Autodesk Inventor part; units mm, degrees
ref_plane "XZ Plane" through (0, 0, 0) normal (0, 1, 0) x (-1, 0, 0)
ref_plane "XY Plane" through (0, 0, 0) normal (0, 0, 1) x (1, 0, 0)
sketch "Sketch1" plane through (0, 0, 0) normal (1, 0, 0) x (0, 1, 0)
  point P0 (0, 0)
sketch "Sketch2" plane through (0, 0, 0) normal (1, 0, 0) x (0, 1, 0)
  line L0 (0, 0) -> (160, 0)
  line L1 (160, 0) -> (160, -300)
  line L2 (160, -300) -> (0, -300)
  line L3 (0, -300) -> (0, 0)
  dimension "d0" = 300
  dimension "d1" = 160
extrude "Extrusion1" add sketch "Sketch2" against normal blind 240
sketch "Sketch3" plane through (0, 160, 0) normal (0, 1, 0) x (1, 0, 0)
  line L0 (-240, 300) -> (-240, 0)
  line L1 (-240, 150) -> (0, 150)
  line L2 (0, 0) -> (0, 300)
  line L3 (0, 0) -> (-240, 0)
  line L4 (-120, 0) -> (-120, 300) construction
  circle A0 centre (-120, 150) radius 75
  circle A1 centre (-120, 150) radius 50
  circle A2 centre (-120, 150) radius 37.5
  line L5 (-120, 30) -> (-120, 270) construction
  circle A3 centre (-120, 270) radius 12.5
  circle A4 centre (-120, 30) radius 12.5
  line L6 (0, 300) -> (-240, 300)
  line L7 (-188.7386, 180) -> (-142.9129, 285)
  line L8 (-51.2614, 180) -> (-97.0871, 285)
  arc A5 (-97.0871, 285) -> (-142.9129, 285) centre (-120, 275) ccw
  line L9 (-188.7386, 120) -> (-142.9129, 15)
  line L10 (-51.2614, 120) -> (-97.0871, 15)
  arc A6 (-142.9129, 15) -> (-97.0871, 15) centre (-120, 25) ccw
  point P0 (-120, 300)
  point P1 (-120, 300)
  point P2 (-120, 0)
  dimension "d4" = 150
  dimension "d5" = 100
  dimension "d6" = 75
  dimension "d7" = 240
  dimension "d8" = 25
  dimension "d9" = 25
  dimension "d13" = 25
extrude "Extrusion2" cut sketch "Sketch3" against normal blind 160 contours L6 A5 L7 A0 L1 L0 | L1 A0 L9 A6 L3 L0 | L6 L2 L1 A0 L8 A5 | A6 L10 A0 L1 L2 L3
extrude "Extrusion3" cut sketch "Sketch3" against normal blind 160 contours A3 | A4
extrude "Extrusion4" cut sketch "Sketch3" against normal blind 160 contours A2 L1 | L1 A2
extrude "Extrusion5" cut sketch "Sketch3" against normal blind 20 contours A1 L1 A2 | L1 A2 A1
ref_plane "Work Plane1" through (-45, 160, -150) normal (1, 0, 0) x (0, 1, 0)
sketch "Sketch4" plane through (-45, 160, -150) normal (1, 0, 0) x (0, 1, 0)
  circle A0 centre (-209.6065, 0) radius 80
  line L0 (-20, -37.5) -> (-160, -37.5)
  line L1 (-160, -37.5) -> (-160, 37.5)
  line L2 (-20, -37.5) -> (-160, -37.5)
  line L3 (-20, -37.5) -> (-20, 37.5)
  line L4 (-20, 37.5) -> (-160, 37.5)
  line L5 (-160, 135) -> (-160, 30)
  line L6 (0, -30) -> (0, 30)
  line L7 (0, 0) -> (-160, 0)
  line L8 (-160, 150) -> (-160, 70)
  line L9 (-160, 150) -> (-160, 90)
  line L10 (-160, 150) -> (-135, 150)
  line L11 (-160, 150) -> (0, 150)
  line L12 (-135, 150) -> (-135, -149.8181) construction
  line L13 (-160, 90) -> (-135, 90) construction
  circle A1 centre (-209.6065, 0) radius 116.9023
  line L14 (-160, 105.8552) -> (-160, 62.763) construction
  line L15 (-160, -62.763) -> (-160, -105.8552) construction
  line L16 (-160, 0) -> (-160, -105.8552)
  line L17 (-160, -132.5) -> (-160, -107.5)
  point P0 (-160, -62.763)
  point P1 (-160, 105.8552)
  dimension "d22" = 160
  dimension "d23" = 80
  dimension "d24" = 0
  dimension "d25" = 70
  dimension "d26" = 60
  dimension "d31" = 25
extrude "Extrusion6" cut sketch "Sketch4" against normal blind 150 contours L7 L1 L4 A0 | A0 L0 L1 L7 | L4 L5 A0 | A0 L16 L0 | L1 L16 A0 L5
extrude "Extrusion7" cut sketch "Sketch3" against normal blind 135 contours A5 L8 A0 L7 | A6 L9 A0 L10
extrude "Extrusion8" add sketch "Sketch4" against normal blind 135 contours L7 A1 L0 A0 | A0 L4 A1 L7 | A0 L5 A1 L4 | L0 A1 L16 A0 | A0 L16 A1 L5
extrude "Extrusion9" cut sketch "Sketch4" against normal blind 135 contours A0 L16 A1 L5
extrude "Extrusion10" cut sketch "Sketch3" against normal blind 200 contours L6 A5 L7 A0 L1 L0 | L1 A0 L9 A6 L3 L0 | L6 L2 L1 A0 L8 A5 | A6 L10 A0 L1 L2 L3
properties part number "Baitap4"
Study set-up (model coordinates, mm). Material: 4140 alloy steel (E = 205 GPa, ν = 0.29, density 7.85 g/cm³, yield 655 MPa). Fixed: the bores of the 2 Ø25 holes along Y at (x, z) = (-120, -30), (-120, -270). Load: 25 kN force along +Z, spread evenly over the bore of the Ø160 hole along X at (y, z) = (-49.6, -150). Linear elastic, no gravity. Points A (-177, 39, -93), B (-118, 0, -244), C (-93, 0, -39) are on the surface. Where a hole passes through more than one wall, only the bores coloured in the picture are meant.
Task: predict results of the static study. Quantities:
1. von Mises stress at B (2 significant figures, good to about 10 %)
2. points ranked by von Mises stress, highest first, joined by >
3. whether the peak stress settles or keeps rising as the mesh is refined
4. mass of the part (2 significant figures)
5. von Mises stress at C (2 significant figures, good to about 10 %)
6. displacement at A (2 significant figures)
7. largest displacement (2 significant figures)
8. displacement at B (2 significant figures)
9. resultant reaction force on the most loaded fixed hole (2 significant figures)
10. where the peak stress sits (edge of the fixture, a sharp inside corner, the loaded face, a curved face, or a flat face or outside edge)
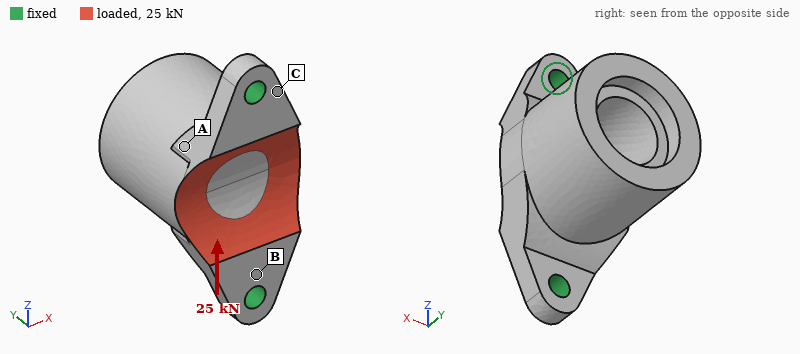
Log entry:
6.8 MPa
B > C > A
keeps rising
18 kg
3.5 MPa
2.8 µm
3.4 µm
0.51 µm
13 kN
edge of the fixture
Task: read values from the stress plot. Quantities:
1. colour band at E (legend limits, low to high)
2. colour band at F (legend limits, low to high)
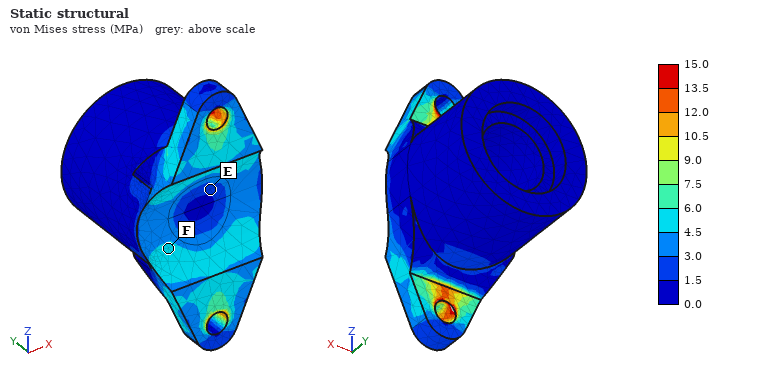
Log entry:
1.5 to 3.0 MPa
4.5 to 6.0 MPa
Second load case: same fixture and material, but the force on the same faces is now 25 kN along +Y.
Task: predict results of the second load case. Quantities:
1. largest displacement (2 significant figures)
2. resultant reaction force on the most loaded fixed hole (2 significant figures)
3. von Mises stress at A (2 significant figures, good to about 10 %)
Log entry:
11 µm
17 kN
5.3 MPa
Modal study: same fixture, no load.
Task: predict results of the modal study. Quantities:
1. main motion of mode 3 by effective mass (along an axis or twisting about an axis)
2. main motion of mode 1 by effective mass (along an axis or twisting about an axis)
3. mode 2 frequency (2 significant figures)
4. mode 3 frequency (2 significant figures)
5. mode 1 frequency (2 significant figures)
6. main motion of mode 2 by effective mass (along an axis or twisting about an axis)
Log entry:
along Z
along X
1900 Hz
2000 Hz
540 Hz
along Y
